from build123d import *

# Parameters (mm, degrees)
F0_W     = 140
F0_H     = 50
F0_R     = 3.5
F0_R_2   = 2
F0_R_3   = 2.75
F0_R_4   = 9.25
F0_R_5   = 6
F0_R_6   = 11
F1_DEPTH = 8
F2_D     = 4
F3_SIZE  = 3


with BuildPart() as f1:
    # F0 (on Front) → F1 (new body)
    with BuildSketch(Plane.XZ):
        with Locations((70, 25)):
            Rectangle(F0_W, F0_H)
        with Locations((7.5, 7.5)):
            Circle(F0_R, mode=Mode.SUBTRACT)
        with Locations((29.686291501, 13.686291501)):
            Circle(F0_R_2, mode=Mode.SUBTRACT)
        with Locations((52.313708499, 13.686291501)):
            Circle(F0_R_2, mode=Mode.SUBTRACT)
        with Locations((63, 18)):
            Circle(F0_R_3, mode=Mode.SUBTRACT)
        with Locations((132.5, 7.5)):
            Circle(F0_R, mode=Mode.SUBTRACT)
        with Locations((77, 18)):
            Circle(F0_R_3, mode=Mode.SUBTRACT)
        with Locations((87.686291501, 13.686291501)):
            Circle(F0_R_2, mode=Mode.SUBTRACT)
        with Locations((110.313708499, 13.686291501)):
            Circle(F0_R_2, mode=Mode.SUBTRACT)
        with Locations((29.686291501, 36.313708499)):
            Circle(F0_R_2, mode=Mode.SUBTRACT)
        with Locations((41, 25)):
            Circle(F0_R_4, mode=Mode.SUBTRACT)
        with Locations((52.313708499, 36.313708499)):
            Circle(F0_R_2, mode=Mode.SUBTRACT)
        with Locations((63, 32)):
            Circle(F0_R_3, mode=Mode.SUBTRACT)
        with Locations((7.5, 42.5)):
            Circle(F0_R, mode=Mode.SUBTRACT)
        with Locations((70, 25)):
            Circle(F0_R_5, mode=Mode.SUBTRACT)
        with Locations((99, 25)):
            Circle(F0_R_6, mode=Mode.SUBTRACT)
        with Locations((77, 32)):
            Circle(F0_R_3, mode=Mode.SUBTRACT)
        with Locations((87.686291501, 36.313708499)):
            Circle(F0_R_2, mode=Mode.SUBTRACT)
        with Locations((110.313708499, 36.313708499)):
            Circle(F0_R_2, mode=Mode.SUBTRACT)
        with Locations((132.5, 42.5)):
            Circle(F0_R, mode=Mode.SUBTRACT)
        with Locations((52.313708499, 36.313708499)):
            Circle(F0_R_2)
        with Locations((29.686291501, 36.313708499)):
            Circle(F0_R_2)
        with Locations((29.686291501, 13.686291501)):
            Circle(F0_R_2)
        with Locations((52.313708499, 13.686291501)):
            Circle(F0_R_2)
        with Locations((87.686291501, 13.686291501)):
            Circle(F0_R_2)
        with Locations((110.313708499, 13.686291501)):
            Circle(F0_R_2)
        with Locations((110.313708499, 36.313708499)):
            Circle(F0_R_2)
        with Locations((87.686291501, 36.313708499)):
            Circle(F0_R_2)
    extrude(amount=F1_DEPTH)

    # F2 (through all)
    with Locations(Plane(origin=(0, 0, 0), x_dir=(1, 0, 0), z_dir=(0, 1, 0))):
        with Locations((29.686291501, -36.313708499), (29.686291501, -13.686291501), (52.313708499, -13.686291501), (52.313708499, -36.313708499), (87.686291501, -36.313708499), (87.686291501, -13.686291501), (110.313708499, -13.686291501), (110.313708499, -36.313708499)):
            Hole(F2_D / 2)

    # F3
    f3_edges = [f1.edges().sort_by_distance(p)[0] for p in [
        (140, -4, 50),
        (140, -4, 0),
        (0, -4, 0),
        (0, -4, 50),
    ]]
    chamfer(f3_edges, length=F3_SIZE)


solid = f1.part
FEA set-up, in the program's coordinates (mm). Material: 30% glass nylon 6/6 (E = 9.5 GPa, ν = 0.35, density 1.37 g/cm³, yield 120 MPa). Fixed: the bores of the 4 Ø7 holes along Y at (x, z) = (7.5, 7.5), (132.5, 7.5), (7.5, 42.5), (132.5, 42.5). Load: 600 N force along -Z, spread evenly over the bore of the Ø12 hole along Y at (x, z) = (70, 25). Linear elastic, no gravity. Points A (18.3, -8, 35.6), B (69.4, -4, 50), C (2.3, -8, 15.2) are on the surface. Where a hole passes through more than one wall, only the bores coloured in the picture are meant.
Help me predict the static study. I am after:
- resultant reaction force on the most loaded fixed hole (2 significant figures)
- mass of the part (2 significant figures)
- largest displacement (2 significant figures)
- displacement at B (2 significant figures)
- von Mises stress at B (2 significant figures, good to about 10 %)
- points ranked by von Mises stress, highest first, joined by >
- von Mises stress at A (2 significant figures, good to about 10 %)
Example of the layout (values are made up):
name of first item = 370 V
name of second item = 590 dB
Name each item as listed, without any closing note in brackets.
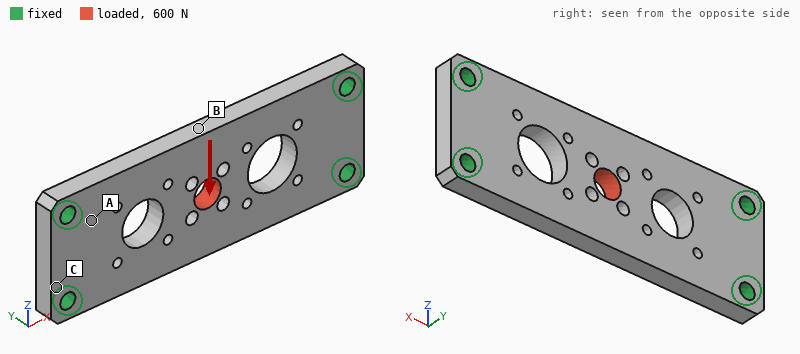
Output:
resultant reaction force on the most loaded fixed hole = 310 N
mass of the part = 64 g
largest displacement = 39 µm
displacement at B = 36 µm
von Mises stress at B = 4.1 MPa
points ranked by von Mises stress, highest first, joined by > = B > A > C
von Mises stress at A = 1.9 MPa
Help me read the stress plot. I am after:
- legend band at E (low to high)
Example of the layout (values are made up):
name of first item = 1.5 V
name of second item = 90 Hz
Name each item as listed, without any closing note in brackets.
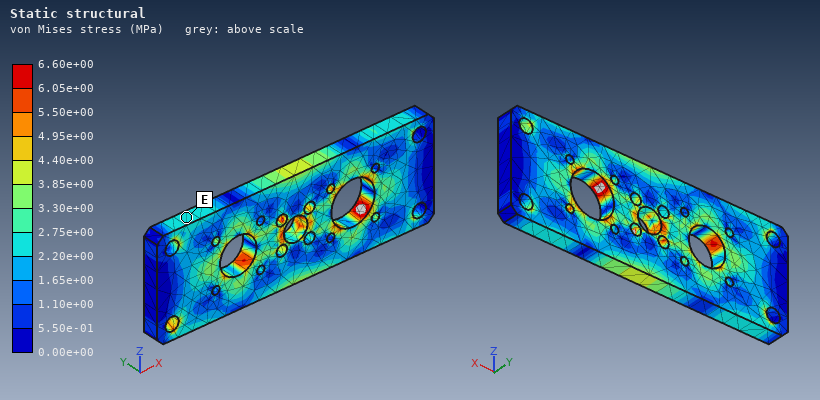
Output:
legend band at E = 2.20e+00 to 2.75e+00 MPa
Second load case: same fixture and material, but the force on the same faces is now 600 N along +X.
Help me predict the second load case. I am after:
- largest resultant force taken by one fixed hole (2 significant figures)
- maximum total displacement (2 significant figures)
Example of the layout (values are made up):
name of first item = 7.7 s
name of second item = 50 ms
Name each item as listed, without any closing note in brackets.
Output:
largest resultant force taken by one fixed hole = 160 N
maximum total displacement = 14 µm
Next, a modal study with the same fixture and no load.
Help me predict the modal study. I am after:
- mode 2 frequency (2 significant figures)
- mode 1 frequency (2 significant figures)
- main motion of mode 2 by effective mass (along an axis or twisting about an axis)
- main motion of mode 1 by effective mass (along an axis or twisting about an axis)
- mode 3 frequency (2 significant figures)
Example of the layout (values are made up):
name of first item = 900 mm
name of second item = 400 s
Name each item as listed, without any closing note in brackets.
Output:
mode 2 frequency = 2300 Hz
mode 1 frequency = 1400 Hz
main motion of mode 2 by effective mass = twisting about X
main motion of mode 1 by effective mass = along Y
mode 3 frequency = 3700 Hz
